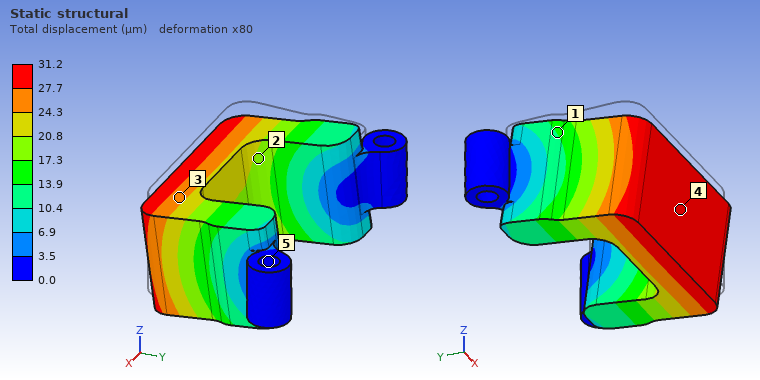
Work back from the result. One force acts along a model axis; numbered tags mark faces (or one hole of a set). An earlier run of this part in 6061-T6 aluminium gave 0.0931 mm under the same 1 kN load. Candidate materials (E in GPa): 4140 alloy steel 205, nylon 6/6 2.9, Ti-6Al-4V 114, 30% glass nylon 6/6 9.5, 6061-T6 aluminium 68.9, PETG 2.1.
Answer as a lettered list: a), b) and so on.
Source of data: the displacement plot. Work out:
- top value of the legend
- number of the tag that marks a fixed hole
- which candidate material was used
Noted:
a) 31.2 µm
b) 5
c) 4140 alloy steel
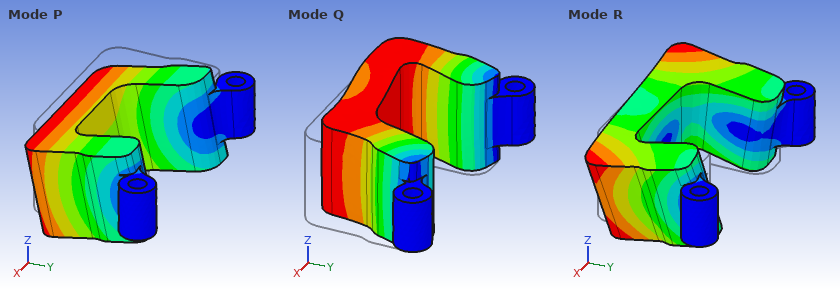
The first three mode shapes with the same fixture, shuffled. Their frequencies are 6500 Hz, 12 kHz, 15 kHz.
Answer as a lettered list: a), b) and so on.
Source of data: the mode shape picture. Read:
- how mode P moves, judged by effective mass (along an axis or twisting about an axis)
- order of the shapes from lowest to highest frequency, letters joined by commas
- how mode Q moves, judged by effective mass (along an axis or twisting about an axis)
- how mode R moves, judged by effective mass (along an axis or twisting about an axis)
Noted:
a) along Z
b) P, Q, R
c) along X
d) twisting about Y
